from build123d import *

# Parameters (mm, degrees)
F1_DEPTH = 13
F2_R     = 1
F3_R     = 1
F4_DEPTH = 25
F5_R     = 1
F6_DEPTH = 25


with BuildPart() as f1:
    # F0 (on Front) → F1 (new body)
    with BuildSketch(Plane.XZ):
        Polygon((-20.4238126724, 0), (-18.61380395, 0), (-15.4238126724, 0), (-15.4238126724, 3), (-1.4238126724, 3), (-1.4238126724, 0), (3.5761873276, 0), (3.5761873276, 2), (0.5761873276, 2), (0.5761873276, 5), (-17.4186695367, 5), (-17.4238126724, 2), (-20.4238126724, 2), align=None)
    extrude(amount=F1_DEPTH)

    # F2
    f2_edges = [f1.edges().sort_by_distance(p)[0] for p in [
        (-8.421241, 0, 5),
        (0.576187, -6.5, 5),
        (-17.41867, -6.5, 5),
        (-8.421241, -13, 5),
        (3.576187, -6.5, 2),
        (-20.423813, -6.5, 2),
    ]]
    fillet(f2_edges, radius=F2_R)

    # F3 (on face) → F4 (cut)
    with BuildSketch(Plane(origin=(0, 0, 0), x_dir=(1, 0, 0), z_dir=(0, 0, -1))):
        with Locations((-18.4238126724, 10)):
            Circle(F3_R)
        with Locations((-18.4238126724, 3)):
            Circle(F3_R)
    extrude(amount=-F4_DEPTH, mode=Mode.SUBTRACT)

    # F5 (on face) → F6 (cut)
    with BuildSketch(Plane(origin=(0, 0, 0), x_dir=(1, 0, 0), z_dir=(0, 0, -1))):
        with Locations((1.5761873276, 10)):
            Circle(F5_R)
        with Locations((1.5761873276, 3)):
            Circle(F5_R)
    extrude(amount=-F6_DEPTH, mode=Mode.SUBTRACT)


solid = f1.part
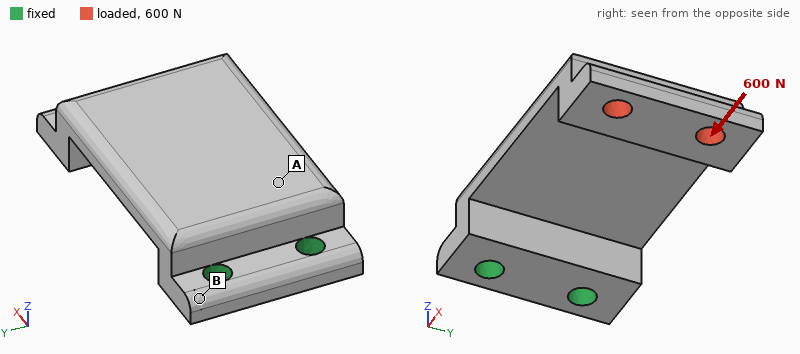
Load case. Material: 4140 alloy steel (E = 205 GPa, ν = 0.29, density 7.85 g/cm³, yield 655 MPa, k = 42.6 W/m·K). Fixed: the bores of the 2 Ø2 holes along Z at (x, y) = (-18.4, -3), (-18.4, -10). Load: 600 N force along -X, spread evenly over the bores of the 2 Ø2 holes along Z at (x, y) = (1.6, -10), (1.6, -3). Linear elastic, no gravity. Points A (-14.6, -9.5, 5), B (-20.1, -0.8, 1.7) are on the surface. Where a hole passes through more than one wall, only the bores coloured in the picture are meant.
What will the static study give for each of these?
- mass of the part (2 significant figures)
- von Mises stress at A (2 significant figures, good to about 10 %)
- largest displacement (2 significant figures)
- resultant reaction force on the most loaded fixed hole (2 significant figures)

5.8 g
170 MPa
0.23 mm
300 N
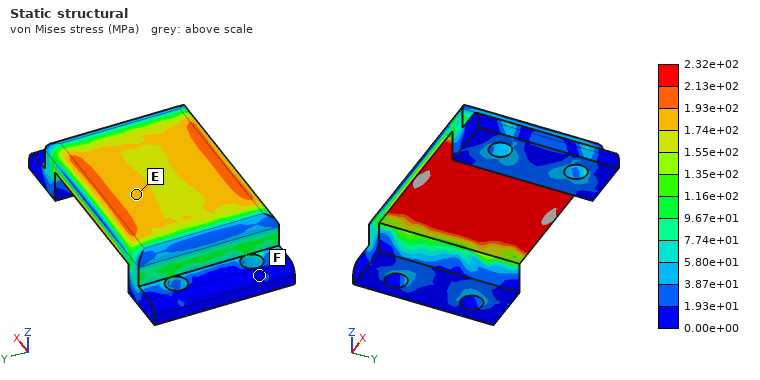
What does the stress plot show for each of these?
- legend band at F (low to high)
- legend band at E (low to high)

0.00e+00 to 1.93e+01 MPa
1.74e+02 to 1.93e+02 MPa
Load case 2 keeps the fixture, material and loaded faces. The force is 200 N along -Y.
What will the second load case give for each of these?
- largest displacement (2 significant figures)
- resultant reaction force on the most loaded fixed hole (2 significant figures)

58 µm
470 N
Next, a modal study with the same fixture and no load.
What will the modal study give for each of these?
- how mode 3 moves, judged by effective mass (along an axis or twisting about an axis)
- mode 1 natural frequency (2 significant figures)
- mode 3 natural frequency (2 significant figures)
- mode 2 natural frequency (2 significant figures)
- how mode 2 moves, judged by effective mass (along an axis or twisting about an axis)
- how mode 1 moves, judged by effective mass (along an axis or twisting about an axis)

along Y
2800 Hz
14 kHz
7800 Hz
along Y
along Z
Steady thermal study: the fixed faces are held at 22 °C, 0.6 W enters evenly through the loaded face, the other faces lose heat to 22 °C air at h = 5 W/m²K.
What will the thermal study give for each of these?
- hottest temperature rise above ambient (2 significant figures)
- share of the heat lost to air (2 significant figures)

13 K
4.3 %
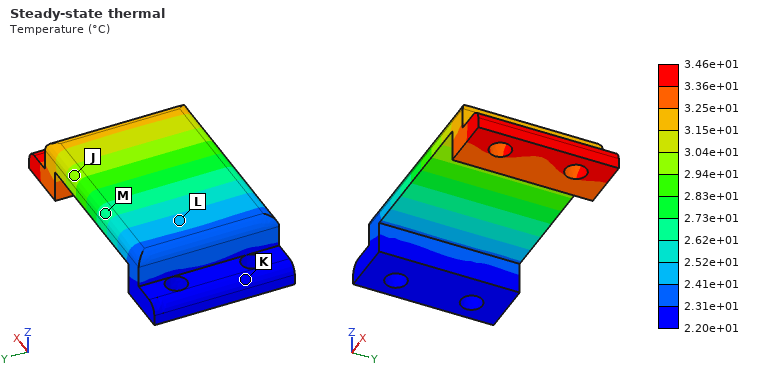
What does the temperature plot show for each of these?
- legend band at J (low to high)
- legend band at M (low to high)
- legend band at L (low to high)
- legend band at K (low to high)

2.94e+01 to 3.04e+01 °C
2.62e+01 to 2.73e+01 °C
2.41e+01 to 2.52e+01 °C
2.20e+01 to 2.31e+01 °C
